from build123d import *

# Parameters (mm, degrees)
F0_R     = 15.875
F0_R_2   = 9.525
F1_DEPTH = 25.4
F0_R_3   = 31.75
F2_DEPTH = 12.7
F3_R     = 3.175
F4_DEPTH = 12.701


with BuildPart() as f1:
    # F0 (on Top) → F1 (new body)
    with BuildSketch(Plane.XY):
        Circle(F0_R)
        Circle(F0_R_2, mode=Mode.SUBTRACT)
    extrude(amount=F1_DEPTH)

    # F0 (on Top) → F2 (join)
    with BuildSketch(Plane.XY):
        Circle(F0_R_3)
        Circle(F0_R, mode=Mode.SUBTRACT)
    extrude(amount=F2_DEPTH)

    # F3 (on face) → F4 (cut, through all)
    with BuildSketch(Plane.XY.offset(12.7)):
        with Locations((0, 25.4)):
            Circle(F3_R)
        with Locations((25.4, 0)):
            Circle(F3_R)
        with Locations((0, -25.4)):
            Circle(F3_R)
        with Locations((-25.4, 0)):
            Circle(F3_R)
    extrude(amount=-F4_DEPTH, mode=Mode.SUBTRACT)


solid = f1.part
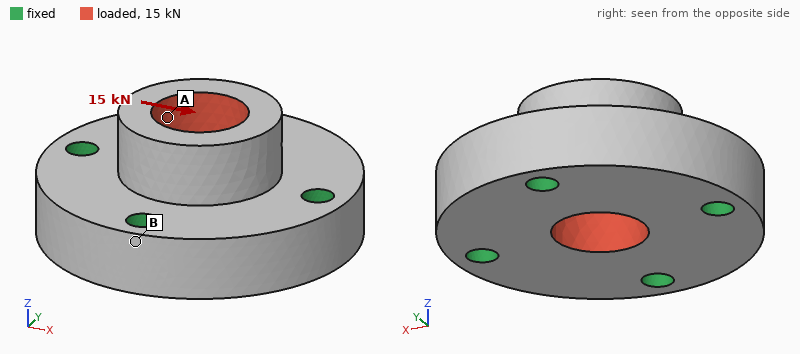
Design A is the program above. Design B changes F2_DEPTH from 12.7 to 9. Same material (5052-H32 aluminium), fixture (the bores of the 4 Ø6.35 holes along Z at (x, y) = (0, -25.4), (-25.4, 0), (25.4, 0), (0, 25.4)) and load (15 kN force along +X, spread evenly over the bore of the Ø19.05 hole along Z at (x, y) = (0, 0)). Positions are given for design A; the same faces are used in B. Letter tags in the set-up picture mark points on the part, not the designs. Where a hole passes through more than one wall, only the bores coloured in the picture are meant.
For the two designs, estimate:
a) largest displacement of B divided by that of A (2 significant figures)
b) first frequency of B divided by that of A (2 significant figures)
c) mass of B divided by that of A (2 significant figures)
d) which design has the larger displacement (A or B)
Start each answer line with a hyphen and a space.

- 1.8
- 0.76
- 0.80
- B
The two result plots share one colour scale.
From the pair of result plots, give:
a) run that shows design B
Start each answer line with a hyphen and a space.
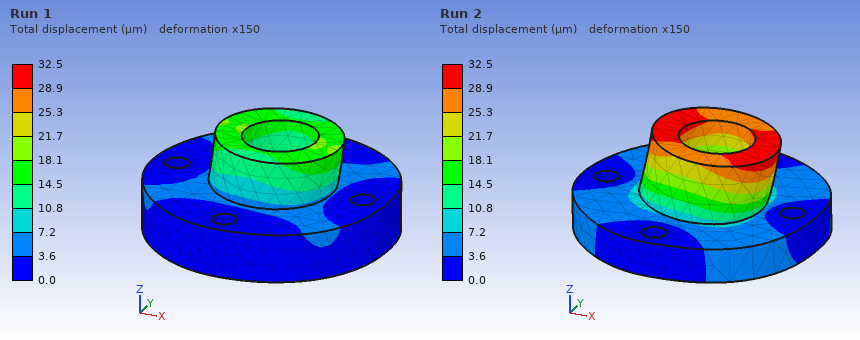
- Run 2
